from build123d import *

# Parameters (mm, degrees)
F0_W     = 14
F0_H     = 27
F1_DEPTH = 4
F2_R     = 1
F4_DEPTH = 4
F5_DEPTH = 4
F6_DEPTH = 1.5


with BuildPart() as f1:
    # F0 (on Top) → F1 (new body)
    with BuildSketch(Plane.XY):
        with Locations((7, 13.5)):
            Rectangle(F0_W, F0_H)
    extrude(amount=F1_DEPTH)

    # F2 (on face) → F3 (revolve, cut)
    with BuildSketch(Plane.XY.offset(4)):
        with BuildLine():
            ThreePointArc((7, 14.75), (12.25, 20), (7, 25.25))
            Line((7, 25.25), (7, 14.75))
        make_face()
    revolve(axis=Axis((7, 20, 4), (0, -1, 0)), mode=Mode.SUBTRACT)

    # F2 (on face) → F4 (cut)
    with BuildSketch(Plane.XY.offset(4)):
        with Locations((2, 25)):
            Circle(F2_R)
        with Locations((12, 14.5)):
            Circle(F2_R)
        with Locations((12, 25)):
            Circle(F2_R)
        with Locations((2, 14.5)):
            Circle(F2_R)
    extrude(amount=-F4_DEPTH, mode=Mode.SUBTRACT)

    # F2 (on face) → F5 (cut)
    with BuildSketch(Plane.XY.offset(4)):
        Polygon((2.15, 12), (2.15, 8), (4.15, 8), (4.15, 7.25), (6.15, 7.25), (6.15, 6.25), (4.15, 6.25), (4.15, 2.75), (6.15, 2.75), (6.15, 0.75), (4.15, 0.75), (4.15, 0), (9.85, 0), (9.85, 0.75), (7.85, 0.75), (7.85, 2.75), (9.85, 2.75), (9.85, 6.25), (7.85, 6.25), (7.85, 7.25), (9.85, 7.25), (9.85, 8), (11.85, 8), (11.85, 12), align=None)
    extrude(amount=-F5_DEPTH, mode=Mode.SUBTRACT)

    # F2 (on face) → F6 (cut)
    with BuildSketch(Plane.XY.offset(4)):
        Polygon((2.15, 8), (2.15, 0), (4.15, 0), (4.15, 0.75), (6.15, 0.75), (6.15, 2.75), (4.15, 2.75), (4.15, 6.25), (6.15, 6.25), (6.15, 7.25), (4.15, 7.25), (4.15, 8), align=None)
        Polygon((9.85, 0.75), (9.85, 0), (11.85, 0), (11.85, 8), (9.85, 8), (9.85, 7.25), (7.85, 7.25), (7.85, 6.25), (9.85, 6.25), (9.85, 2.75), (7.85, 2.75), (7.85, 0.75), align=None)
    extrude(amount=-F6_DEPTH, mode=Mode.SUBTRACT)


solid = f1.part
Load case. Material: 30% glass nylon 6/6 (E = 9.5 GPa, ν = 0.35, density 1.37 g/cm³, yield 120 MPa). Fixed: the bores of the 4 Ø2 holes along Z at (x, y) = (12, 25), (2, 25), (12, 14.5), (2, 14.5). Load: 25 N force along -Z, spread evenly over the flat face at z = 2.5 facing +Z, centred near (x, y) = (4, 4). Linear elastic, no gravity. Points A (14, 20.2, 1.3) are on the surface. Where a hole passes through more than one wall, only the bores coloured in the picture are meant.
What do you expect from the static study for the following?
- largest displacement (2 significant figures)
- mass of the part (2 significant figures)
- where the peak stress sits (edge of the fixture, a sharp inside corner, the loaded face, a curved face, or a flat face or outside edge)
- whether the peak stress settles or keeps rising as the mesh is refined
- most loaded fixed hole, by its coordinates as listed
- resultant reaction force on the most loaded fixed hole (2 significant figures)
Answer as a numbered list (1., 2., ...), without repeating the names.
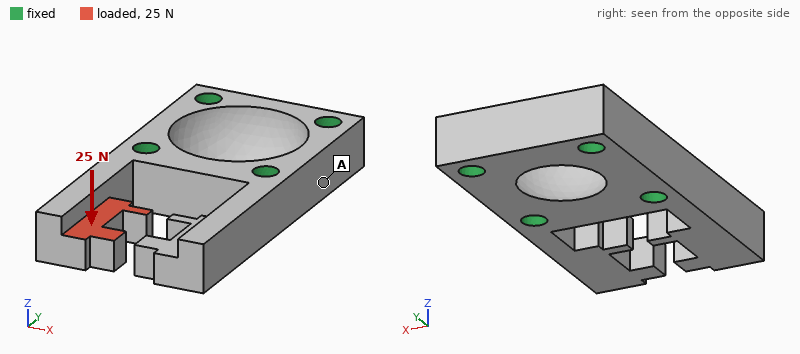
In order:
1. 0.19 mm
2. 1.1 g
3. edge of the fixture
4. keeps rising
5. (2, 14.5)
6. 25 N
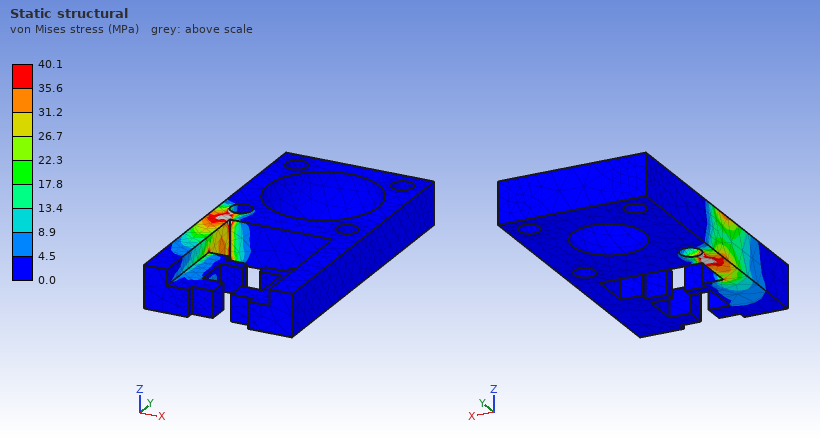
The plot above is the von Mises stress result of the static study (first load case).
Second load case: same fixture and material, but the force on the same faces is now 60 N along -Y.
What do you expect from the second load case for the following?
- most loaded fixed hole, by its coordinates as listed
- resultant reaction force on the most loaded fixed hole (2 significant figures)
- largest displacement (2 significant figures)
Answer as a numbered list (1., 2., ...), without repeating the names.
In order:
1. (2, 14.5)
2. 58 N
3. 0.34 mm
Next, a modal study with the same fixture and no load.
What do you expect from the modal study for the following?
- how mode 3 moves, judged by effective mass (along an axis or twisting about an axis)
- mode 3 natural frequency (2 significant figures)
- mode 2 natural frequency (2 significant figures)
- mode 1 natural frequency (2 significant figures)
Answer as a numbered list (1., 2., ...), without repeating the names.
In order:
1. along Z
2. 6100 Hz
3. 3900 Hz
4. 3900 Hz
